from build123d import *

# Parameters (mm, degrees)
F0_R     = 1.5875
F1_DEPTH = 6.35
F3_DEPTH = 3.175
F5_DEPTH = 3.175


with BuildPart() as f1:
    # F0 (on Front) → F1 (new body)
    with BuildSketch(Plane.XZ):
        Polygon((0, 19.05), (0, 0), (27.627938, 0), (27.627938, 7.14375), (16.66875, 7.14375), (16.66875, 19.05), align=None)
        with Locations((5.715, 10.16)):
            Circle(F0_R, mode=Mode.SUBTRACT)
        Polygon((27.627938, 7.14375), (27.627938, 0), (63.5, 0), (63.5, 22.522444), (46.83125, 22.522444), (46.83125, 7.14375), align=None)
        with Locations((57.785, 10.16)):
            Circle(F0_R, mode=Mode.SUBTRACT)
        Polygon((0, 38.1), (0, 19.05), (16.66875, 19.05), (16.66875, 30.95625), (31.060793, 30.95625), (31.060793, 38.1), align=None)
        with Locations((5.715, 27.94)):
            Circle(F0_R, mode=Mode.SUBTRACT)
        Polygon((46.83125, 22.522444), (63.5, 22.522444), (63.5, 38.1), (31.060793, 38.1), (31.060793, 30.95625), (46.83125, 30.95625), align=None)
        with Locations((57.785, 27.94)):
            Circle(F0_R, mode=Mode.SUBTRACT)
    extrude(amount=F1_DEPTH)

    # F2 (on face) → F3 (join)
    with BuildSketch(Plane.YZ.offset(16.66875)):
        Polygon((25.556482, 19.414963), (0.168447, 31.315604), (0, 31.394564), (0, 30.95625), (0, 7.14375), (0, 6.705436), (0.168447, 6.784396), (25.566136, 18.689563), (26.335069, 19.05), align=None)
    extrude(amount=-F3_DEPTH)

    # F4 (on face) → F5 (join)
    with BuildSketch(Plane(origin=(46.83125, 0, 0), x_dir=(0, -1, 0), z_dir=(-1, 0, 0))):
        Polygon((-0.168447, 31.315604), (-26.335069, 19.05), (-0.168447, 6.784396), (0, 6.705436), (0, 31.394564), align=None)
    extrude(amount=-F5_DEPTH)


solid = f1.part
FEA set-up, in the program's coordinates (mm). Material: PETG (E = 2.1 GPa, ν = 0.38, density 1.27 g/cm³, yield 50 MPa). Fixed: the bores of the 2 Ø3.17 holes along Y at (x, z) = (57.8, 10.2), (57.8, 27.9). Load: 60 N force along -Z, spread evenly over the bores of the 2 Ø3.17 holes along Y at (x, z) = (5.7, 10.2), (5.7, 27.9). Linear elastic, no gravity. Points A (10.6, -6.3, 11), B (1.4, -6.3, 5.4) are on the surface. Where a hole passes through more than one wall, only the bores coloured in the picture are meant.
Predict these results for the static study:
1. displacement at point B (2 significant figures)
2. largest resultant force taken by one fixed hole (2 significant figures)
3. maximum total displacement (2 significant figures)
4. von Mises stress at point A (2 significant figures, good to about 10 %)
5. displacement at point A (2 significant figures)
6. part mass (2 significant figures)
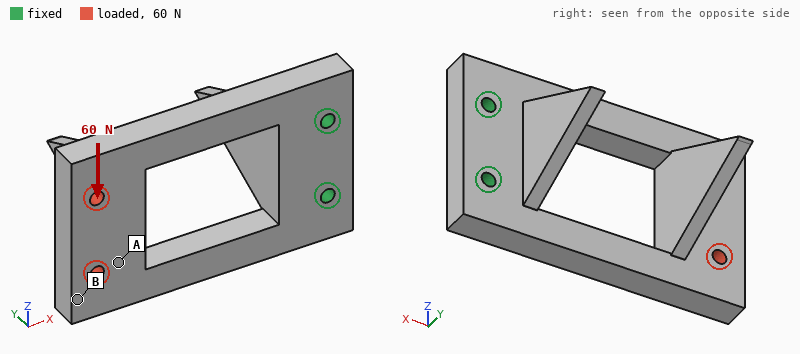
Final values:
0.53 mm
150 N
0.54 mm
1.9 MPa
0.50 mm
16 g
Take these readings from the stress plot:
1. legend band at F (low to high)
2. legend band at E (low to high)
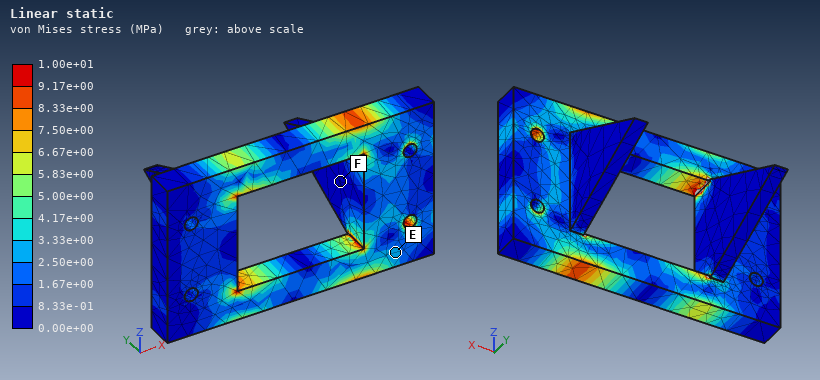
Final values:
0.00e+00 to 8.33e-01 MPa
2.50e+00 to 3.33e+00 MPa
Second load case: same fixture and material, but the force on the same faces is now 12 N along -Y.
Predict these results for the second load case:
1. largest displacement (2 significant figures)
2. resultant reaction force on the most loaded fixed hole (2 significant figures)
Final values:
0.87 mm
6.2 N
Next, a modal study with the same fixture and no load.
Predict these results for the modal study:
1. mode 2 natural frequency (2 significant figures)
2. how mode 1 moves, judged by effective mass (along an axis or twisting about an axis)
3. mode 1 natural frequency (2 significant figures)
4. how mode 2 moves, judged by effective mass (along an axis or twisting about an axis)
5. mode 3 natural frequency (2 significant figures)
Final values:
630 Hz
along Y
270 Hz
along Z
780 Hz
